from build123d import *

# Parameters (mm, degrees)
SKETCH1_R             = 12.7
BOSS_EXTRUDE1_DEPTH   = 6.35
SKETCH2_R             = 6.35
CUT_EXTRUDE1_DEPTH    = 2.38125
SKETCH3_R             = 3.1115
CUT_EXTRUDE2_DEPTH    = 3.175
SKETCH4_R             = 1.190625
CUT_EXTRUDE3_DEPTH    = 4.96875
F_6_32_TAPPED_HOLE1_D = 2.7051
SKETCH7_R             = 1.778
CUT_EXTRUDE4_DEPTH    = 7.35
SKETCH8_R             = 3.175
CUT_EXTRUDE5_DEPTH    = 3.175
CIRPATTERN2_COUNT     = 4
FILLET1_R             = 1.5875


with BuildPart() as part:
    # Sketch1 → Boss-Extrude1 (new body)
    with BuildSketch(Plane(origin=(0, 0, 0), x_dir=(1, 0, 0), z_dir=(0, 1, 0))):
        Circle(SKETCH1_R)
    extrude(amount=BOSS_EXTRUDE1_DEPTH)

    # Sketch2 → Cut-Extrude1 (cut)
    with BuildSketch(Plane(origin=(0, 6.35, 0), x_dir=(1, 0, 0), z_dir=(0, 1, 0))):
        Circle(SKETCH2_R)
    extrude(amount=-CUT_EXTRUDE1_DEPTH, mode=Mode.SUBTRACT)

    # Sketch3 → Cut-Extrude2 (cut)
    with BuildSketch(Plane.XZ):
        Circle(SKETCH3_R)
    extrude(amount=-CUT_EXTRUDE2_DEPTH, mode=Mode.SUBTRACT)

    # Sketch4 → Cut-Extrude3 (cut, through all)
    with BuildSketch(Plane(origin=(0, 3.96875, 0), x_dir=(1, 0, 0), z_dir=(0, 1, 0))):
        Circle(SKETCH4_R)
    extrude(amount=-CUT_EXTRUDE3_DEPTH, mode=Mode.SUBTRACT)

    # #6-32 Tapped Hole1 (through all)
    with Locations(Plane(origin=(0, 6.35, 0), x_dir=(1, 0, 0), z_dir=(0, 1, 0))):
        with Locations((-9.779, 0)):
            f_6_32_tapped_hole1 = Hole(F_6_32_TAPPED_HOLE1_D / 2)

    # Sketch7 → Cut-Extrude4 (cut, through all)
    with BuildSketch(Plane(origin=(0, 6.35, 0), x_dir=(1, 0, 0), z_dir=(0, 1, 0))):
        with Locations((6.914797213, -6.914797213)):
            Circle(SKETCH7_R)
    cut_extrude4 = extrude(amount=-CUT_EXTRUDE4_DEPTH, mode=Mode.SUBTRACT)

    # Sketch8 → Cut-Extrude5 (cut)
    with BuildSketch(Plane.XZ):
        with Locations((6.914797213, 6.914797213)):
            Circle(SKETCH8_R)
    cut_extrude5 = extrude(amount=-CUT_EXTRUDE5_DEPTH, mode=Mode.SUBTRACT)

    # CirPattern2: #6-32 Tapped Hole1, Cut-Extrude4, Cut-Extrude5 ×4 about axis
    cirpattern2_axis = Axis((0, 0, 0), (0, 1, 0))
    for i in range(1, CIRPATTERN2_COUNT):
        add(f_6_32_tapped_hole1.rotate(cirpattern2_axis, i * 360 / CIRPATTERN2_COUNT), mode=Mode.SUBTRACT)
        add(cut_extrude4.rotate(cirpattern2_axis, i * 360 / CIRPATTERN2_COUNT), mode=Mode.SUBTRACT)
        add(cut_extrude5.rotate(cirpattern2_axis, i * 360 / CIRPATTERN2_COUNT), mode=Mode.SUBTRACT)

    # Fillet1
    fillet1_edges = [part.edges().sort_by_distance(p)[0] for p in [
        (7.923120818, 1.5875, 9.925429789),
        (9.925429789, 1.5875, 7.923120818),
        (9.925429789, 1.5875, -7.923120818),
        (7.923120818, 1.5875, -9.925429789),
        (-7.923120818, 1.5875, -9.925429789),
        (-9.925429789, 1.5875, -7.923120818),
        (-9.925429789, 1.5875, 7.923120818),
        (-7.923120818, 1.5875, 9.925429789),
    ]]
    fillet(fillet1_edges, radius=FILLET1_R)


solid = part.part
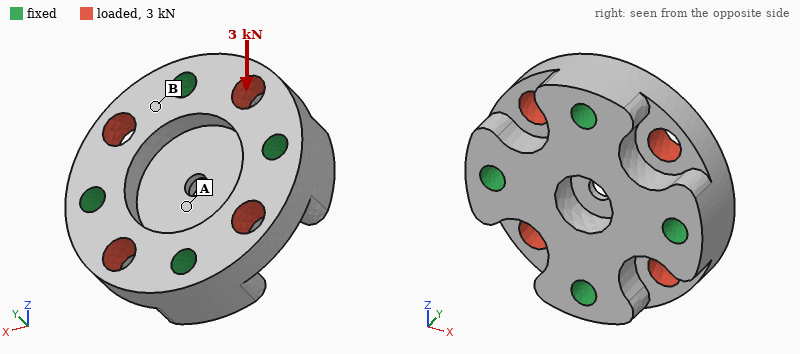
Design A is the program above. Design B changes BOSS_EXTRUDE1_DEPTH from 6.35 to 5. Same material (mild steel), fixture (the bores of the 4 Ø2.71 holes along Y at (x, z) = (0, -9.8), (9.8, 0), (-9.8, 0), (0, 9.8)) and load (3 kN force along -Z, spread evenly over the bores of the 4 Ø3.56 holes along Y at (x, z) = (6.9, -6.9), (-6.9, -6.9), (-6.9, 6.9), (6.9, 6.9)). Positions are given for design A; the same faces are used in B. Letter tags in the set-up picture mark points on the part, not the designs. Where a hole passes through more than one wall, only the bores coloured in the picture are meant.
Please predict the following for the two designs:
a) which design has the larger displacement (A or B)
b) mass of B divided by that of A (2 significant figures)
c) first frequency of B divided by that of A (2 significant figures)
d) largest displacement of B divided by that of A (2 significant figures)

B
0.79
0.92
1.5
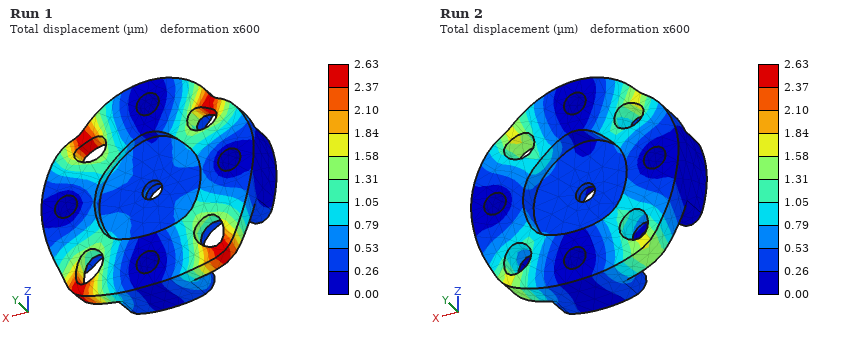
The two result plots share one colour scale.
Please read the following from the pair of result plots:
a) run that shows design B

Run 1
